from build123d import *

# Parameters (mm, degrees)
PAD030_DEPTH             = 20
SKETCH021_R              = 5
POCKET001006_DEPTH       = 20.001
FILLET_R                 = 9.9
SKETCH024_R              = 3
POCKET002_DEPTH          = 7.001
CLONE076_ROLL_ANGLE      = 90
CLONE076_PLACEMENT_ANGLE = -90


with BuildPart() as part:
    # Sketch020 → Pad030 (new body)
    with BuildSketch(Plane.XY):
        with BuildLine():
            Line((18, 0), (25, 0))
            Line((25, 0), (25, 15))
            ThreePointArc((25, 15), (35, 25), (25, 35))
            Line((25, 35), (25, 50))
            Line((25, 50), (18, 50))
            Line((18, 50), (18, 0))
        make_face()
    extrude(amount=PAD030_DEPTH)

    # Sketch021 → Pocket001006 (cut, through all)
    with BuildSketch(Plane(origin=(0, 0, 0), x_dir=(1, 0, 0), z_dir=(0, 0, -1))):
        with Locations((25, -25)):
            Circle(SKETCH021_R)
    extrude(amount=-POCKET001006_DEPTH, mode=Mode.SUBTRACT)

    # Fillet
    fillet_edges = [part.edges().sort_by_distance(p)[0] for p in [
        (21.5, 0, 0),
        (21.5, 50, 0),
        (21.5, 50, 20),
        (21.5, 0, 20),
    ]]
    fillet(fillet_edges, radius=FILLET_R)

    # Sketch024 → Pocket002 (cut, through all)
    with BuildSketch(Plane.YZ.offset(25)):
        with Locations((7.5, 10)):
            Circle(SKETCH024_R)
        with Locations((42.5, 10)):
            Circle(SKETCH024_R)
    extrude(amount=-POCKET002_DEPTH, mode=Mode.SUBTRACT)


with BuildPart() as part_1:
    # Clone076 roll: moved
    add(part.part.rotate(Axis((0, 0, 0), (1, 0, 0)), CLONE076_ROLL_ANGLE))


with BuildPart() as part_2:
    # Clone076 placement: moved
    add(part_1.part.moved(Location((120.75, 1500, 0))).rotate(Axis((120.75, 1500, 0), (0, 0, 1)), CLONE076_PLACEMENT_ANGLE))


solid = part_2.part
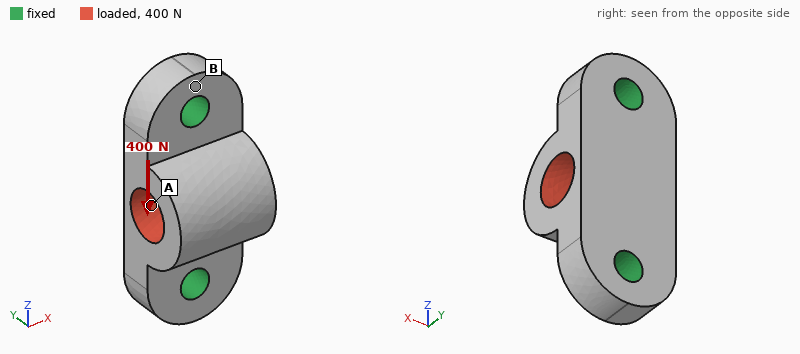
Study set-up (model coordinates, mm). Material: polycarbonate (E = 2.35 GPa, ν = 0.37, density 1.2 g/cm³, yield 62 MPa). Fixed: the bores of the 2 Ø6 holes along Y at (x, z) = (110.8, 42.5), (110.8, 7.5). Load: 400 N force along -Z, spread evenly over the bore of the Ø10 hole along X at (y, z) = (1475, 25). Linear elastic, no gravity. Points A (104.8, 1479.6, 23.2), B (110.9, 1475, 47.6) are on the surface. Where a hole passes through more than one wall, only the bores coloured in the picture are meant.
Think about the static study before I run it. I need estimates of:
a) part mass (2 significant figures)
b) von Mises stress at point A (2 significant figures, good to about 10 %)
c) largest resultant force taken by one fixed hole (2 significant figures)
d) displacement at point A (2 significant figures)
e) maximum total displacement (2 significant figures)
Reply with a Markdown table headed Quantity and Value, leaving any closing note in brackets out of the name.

| Quantity | Value |
|---|---|
| part mass | 9.1 g |
| von Mises stress at point A | 1.3 MPa |
| largest resultant force taken by one fixed hole | 200 N |
| displacement at point A | 7.7 µm |
| maximum total displacement | 22 µm |
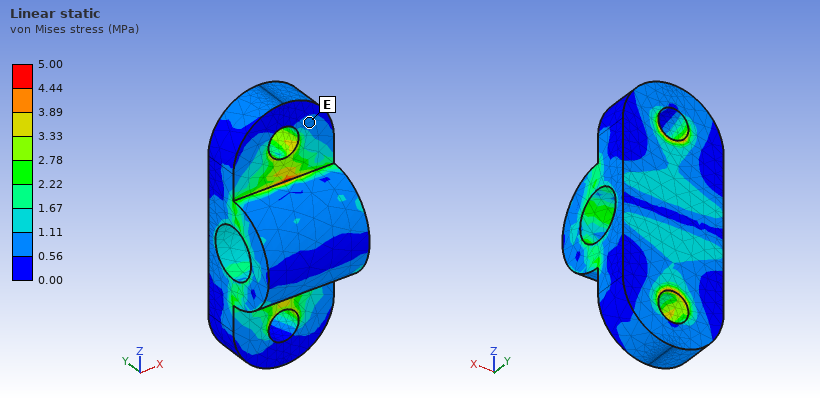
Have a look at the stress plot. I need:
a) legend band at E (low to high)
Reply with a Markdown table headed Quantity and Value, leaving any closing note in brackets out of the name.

| Quantity | Value |
|---|---|
| legend band at E | 0.56 to 1.11 MPa |
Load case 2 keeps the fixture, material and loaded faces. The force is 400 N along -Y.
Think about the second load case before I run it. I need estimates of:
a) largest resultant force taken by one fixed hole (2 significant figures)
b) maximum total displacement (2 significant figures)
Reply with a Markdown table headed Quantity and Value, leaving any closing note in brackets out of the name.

| Quantity | Value |
|---|---|
| largest resultant force taken by one fixed hole | 200 N |
| maximum total displacement | 57 µm |
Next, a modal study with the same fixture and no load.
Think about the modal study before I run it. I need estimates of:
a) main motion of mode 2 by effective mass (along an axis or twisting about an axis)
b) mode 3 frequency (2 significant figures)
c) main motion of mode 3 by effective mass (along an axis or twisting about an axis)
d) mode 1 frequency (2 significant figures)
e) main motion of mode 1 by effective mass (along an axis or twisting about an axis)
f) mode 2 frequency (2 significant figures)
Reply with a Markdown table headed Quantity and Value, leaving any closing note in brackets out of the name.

| Quantity | Value |
|---|---|
| main motion of mode 2 by effective mass | along Y |
| mode 3 frequency | 8700 Hz |
| main motion of mode 3 by effective mass | along X |
| mode 1 frequency | 4700 Hz |
| main motion of mode 1 by effective mass | along X |
| mode 2 frequency | 7100 Hz |
